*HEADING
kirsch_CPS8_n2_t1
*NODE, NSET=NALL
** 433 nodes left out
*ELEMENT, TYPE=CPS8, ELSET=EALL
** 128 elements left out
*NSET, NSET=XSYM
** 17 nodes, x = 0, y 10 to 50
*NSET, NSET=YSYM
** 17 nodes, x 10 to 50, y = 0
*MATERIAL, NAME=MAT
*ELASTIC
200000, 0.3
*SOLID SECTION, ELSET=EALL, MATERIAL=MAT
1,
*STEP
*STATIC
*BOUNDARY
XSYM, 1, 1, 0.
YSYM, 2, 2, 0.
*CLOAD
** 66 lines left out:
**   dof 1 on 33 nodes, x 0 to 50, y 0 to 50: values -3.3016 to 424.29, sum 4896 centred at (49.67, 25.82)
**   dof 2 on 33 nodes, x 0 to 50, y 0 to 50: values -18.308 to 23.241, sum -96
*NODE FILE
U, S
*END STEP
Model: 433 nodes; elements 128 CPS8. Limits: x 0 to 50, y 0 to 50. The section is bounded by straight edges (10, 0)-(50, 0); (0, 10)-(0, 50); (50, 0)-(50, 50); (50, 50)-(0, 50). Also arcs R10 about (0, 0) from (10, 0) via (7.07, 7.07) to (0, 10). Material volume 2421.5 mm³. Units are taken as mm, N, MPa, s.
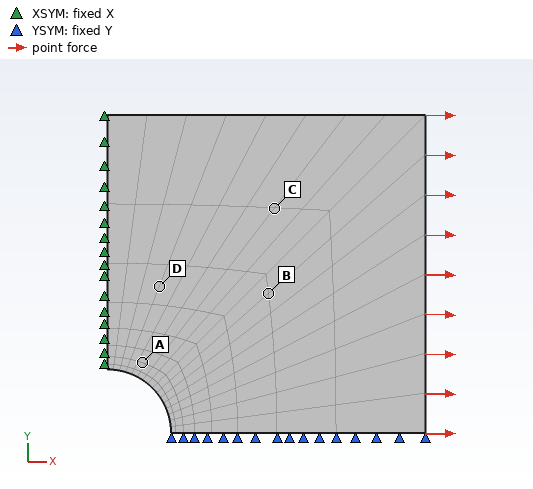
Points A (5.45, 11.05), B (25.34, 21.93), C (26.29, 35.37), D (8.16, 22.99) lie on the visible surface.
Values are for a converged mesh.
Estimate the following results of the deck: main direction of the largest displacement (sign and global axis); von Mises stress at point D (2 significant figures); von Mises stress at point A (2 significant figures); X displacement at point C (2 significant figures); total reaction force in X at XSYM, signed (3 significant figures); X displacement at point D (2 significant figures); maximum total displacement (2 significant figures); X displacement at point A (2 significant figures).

+X
110 MPa
160 MPa
0.014 mm
-4900 N
0.0045 mm
0.029 mm
0.0054 mm
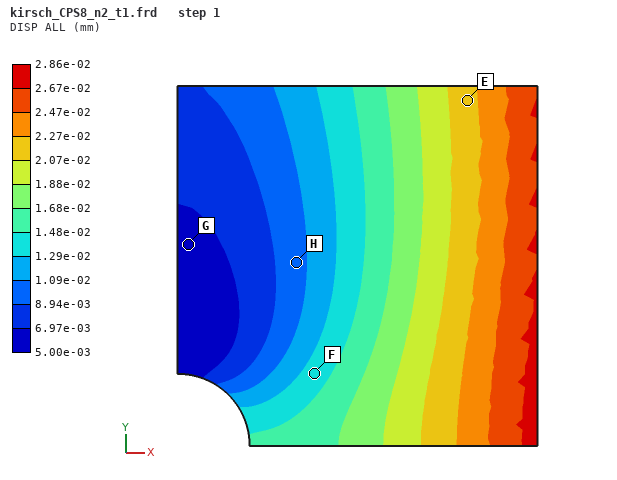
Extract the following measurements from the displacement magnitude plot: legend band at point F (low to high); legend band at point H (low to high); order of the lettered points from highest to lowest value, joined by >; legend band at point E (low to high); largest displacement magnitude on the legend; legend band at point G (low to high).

1.29e-02 to 1.48e-02 mm
8.94e-03 to 1.09e-02 mm
E > F > H > G
2.07e-02 to 2.27e-02 mm
2.86e-02 mm
5.00e-03 to 6.97e-03 mm
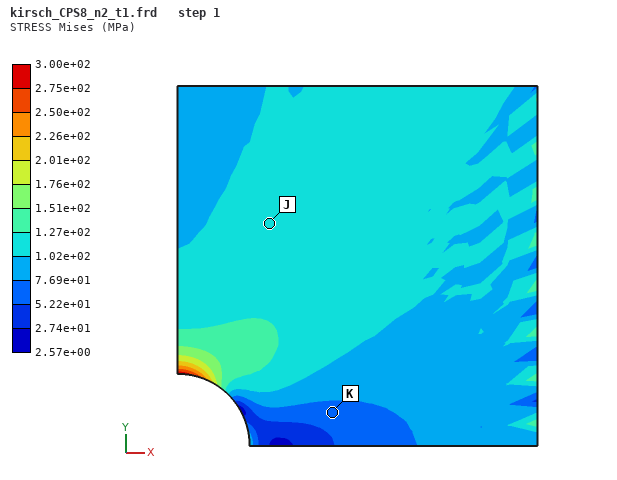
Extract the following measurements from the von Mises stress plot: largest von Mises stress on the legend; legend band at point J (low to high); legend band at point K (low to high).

3.00e+02 MPa
1.02e+02 to 1.27e+02 MPa
5.22e+01 to 7.69e+01 MPa
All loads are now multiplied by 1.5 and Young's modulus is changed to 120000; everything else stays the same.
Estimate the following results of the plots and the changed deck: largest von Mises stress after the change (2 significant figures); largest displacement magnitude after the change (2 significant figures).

450 MPa
0.072 mm
